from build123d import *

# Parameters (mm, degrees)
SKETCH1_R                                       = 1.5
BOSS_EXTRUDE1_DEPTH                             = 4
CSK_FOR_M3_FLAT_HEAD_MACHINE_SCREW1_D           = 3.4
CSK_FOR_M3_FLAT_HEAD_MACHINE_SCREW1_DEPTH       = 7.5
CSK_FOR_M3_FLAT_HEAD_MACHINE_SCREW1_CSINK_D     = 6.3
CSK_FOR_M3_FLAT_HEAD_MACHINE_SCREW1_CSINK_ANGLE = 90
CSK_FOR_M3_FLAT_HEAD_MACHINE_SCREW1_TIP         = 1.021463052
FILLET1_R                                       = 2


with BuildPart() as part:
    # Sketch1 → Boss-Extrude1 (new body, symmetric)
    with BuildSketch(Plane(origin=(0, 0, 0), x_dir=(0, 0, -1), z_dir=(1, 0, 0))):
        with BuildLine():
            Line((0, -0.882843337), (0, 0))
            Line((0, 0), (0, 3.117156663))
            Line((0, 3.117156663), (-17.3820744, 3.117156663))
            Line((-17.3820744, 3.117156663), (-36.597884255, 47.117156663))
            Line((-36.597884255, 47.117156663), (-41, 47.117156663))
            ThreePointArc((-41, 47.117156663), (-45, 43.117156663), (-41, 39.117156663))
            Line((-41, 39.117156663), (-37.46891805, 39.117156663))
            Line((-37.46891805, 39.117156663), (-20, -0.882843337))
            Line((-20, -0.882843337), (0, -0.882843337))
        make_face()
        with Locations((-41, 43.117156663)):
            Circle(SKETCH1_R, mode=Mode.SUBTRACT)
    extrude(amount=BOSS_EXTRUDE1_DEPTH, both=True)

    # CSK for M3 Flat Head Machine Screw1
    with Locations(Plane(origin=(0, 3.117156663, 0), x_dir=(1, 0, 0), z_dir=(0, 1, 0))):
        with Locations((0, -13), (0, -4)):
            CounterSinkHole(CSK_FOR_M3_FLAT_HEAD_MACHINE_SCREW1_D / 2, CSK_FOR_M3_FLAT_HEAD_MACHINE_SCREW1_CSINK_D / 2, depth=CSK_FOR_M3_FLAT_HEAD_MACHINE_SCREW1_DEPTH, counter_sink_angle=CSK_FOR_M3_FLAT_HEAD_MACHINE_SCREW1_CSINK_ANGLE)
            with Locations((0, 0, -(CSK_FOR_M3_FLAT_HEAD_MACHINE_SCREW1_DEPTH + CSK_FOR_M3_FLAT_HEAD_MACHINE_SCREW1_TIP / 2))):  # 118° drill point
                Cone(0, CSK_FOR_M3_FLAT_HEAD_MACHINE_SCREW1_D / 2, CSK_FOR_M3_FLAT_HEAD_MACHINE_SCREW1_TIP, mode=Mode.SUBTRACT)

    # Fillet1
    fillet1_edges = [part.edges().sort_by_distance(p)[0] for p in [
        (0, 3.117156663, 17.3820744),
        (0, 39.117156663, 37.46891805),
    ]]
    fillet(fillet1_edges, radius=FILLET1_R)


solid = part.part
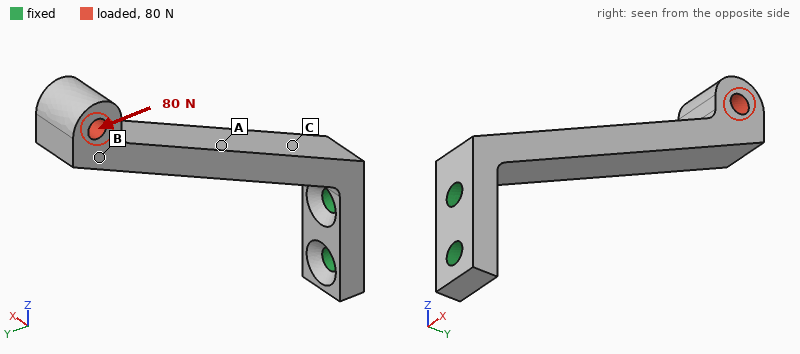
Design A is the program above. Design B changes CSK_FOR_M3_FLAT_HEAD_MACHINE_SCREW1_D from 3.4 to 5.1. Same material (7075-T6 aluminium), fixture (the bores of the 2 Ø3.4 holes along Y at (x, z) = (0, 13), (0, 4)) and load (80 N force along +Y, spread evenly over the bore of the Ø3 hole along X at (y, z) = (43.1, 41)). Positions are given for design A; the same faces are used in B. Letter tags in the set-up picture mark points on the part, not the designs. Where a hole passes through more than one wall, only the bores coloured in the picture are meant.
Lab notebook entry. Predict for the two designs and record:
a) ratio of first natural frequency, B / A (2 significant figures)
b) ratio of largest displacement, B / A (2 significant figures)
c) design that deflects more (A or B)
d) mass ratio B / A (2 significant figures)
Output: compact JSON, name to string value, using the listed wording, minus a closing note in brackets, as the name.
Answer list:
{"ratio of first natural frequency, B / A": "1.1", "ratio of largest displacement, B / A": "0.87", "design that deflects more": "A", "mass ratio B / A": "0.97"}
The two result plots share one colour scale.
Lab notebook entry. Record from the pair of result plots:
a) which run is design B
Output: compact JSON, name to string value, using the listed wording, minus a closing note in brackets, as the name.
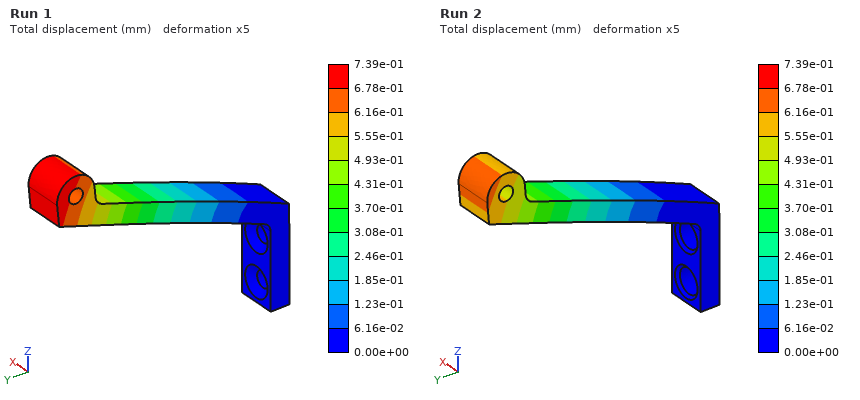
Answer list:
{"which run is design B": "Run 2"}
